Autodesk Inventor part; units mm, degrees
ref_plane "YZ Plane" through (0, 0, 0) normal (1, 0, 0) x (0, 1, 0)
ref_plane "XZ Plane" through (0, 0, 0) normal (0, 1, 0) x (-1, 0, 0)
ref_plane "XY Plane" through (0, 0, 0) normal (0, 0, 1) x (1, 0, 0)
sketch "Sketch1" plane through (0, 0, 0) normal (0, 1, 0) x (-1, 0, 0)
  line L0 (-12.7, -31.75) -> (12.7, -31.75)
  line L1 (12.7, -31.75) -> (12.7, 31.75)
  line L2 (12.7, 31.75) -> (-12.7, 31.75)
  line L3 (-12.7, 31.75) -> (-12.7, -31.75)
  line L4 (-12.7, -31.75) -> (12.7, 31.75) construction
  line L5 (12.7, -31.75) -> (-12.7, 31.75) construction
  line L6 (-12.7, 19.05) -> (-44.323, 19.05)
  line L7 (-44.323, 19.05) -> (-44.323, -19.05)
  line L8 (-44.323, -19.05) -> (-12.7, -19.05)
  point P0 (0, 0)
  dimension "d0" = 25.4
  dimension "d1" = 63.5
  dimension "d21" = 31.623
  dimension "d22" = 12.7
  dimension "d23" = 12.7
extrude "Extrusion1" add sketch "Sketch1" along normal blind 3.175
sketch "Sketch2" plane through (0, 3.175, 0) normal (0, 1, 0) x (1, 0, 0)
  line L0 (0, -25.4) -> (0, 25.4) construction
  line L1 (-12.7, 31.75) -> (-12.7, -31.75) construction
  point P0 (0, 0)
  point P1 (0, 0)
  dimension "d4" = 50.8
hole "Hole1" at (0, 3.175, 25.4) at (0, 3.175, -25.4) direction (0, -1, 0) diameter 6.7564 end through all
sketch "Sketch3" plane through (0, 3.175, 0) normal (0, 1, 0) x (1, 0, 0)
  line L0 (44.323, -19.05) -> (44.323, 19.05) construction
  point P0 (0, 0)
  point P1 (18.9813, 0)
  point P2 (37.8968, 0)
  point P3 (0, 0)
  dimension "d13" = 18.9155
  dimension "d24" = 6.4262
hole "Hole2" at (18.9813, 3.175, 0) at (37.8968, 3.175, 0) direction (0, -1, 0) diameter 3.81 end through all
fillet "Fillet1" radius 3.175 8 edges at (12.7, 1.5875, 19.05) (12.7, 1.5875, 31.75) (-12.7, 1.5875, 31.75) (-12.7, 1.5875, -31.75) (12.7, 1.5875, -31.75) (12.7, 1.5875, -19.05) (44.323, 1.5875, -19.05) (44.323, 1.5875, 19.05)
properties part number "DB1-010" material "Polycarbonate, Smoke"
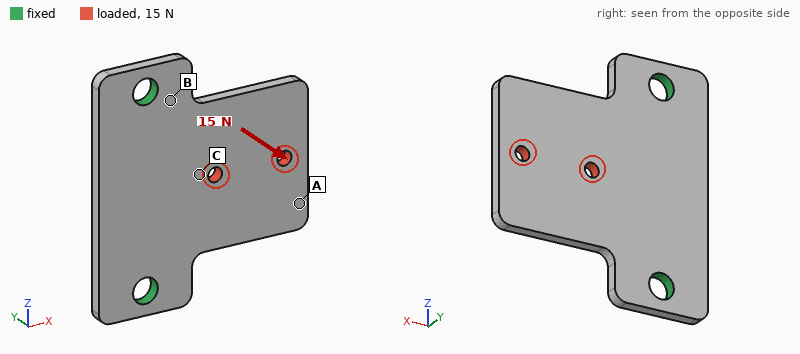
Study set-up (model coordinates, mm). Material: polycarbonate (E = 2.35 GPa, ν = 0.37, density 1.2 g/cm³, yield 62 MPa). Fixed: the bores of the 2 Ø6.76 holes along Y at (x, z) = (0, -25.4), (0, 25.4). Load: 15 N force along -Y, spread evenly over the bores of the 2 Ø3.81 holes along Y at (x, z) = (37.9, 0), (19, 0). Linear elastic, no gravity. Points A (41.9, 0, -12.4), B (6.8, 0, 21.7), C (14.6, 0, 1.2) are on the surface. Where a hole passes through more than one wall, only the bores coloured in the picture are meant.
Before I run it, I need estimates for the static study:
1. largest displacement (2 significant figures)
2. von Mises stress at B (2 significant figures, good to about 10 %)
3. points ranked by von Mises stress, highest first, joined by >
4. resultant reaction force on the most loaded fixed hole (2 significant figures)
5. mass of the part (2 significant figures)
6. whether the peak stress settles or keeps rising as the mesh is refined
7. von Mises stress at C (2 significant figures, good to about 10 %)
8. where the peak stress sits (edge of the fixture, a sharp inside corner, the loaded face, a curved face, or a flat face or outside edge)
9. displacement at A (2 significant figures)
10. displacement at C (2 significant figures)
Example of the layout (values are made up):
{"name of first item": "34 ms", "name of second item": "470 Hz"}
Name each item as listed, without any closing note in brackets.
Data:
{"largest displacement": "1.00 mm", "von Mises stress at B": "4.7 MPa", "points ranked by von Mises stress, highest first, joined by >": "B > C > A", "resultant reaction force on the most loaded fixed hole": "7.5 N", "mass of the part": "10 g", "whether the peak stress settles or keeps rising as the mesh is refined": "keeps rising", "von Mises stress at C": "2.9 MPa", "where the peak stress sits": "edge of the fixture", "displacement at A": "0.89 mm", "displacement at C": "0.23 mm"}
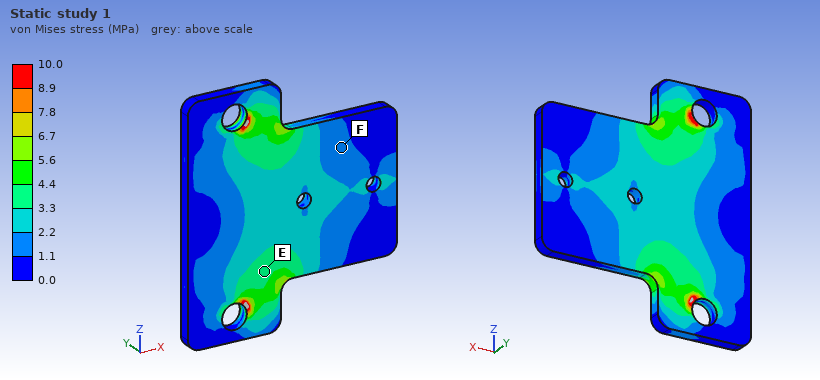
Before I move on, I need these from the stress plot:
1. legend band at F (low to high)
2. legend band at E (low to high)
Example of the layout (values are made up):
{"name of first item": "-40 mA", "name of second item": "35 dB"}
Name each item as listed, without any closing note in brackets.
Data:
{"legend band at F": "1.1 to 2.2 MPa", "legend band at E": "3.3 to 4.4 MPa"}
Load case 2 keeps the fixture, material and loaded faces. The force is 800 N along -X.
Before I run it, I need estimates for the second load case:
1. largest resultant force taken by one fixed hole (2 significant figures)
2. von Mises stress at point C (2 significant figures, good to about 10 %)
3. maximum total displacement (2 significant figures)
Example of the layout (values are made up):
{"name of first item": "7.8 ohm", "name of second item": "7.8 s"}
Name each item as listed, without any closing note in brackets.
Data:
{"largest resultant force taken by one fixed hole": "430 N", "von Mises stress at point C": "8.0 MPa", "maximum total displacement": "0.19 mm"}
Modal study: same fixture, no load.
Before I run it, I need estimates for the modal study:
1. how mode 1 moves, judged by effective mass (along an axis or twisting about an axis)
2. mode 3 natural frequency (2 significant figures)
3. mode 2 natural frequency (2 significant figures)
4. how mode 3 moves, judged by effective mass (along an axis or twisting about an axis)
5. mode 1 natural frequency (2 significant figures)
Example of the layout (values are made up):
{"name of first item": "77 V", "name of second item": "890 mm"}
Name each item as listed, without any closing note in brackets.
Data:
{"how mode 1 moves, judged by effective mass": "along Y", "mode 3 natural frequency": "1800 Hz", "mode 2 natural frequency": "1100 Hz", "how mode 3 moves, judged by effective mass": "along Y", "mode 1 natural frequency": "370 Hz"}
